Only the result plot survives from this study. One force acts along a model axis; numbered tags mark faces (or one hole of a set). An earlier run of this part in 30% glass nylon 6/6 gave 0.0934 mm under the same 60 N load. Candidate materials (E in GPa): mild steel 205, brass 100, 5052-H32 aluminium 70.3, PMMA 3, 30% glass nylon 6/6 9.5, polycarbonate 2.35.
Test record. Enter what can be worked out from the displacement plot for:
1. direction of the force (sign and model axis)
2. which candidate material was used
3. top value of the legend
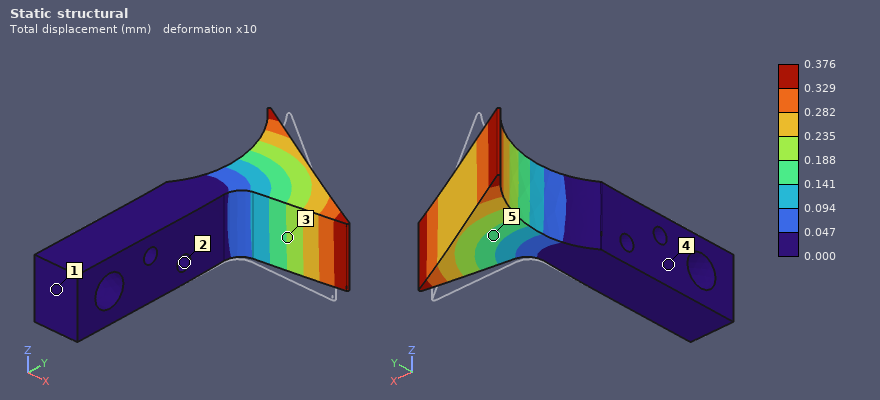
+Y
polycarbonate
0.376 mm
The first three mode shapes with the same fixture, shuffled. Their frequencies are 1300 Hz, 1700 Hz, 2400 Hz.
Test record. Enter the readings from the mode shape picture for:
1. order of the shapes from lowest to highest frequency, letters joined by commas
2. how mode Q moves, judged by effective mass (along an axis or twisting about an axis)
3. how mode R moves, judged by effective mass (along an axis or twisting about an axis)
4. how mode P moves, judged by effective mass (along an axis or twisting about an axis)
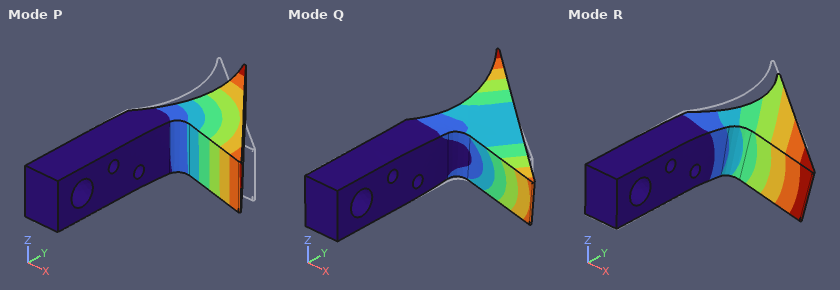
P, R, Q
twisting about Y
along Z
along X
